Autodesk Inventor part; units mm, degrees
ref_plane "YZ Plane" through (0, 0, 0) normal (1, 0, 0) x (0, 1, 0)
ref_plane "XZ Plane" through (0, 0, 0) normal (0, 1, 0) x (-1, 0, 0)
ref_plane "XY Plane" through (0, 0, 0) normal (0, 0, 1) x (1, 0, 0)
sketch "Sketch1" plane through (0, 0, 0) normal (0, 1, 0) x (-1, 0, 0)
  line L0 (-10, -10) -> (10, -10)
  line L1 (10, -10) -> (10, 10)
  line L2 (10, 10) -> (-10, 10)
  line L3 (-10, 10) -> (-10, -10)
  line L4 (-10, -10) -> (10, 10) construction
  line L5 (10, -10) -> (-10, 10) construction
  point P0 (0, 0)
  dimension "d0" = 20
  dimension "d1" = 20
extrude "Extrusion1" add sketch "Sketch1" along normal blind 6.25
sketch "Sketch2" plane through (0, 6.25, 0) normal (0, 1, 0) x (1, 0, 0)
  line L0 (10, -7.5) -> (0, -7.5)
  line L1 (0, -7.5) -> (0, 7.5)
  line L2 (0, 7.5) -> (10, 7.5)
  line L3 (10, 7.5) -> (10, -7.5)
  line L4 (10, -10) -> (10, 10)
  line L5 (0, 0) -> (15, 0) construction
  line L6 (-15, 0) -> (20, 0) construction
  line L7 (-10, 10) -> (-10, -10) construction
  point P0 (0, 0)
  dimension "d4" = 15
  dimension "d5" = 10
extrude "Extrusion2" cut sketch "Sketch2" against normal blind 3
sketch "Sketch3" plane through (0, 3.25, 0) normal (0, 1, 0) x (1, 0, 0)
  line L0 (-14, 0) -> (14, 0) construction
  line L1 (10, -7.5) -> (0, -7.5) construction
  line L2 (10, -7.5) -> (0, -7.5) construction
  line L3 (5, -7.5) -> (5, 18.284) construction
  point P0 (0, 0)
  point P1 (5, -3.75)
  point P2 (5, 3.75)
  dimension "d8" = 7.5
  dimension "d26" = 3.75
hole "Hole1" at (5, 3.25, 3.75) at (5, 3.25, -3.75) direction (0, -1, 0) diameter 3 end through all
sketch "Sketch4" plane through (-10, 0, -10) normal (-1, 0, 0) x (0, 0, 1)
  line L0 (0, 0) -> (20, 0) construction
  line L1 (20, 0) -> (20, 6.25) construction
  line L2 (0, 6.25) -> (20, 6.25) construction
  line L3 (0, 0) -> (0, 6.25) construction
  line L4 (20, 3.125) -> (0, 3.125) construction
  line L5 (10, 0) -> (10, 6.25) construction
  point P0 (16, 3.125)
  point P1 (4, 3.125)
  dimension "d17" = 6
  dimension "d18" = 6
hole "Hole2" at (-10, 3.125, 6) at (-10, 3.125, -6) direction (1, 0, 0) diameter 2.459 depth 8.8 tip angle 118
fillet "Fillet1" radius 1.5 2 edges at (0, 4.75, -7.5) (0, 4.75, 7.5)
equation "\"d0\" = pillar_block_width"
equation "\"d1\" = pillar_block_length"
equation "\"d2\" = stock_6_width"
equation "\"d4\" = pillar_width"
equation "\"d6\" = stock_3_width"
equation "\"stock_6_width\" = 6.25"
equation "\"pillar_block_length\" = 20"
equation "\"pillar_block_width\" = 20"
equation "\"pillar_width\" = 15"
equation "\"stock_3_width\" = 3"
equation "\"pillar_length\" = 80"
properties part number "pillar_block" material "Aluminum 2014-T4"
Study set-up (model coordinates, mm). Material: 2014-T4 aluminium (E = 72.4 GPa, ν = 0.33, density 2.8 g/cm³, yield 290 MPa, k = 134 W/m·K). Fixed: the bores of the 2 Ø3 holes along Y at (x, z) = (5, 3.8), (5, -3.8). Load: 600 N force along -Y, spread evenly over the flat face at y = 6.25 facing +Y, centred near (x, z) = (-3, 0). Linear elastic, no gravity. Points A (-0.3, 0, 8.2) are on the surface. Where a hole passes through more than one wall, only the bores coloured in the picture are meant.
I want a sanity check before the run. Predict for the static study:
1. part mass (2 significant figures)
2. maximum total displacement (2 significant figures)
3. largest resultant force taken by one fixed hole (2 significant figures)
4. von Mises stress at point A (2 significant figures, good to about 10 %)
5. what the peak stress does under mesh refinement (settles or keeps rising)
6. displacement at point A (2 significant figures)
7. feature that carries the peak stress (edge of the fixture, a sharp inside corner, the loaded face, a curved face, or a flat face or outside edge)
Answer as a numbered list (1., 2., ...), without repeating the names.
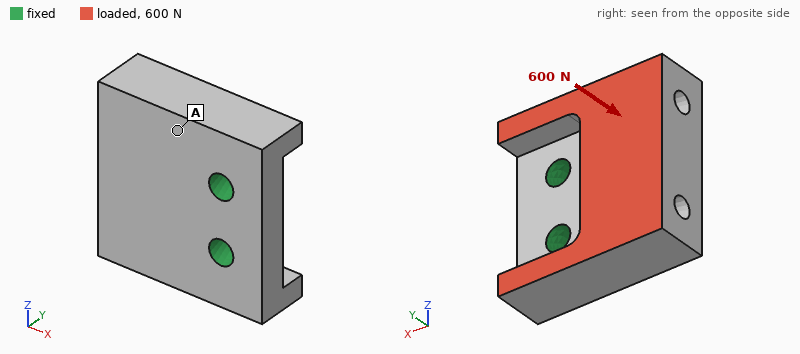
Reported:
1. 5.4 g
2. 43 µm
3. 300 N
4. 28 MPa
5. keeps rising
6. 12 µm
7. edge of the fixture
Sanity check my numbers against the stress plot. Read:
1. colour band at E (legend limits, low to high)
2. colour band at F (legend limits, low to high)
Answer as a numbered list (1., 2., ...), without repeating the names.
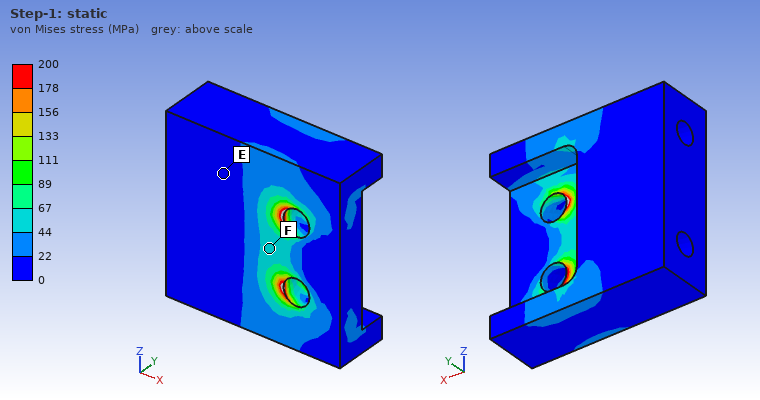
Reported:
1. 0 to 22 MPa
2. 44 to 67 MPa
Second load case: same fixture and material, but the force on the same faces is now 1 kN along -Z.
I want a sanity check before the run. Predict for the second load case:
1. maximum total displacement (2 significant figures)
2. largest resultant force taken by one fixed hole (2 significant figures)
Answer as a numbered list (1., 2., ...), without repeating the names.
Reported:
1. 25 µm
2. 960 N
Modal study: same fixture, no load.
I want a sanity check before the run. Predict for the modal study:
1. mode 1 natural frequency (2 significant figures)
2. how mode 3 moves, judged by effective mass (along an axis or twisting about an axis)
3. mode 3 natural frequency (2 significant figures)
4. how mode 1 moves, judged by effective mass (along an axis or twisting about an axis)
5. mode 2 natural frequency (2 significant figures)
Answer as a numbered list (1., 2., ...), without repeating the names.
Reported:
1. 11 kHz
2. along Z
3. 24 kHz
4. along Y
5. 21 kHz
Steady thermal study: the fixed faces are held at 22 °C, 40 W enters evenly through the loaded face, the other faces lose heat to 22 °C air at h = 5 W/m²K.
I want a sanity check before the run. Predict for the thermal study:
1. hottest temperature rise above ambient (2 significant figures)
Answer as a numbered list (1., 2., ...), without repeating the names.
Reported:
1. 35 K
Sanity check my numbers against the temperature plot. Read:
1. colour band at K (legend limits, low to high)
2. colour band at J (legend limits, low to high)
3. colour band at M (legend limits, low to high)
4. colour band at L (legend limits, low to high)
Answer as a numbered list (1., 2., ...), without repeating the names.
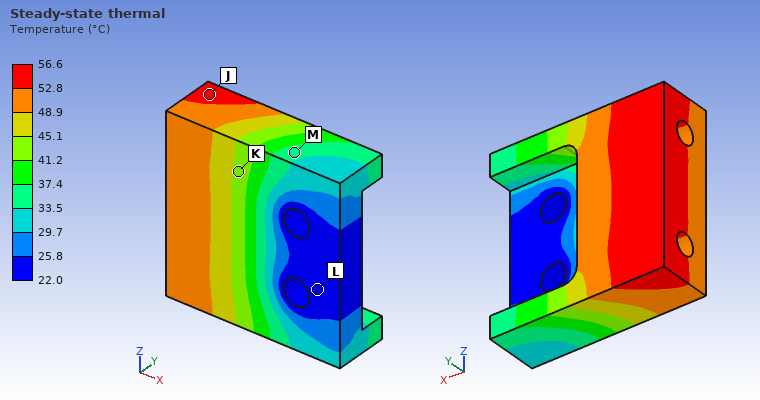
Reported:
1. 41.2 to 45.1 °C
2. 52.8 to 56.6 °C
3. 33.5 to 37.4 °C
4. 22.0 to 25.8 °C
